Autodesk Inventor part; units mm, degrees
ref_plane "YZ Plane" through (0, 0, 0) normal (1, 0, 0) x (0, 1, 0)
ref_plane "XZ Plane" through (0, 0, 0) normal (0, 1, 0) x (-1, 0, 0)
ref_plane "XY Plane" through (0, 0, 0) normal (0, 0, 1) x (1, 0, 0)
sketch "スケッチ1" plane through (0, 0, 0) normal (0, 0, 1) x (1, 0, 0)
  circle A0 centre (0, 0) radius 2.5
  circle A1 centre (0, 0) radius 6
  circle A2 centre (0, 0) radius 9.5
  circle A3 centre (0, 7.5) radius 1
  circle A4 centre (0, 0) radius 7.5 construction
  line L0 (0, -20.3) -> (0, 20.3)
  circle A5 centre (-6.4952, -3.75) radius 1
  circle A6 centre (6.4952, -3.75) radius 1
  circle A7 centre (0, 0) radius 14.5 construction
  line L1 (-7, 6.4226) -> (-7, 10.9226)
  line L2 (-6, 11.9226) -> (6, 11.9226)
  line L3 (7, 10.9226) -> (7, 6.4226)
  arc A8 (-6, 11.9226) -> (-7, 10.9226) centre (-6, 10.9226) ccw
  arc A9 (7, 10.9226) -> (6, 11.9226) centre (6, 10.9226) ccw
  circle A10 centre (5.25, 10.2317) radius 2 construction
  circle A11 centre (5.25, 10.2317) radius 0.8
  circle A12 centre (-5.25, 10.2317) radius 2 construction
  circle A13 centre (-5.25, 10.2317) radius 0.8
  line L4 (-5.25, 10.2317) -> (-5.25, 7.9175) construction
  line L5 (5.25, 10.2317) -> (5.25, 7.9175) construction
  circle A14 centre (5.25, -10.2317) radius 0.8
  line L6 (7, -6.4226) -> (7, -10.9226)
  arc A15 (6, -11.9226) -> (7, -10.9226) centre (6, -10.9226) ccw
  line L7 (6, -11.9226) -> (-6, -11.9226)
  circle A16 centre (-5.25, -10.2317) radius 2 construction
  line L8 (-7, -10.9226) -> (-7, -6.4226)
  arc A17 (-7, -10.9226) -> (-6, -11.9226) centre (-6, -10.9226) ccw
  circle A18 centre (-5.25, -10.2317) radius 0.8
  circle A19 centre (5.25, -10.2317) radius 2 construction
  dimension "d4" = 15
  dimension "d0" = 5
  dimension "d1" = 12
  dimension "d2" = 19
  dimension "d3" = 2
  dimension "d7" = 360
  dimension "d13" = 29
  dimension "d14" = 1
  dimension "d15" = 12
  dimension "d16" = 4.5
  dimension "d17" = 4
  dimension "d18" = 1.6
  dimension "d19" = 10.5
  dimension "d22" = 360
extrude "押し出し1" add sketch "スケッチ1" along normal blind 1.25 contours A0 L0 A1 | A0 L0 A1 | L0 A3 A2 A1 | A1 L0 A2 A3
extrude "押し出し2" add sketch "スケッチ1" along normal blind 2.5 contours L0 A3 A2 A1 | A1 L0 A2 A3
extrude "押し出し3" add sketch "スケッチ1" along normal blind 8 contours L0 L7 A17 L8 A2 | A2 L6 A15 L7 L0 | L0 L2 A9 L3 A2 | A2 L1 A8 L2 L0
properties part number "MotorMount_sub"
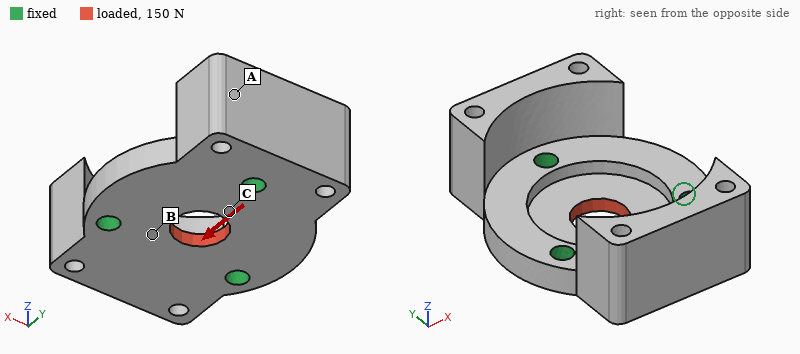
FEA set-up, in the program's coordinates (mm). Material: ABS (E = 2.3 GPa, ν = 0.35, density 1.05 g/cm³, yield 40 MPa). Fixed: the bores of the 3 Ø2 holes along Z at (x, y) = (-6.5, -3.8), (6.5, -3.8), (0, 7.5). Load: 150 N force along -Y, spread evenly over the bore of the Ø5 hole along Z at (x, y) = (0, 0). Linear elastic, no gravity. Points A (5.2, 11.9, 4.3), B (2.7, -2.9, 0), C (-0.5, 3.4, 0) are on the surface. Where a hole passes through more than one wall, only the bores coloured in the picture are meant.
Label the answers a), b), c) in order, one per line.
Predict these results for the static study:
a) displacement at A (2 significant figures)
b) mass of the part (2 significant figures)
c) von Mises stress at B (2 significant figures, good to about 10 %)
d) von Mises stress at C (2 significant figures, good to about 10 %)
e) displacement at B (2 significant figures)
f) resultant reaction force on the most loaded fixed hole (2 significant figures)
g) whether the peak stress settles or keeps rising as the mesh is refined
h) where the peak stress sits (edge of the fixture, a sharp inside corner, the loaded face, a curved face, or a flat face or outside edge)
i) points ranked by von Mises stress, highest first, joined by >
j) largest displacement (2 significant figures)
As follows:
a) 4.1 µm
b) 1.3 g
c) 5.2 MPa
d) 8.5 MPa
e) 15 µm
f) 51 N
g) keeps rising
h) edge of the fixture
i) C > B > A
j) 26 µm
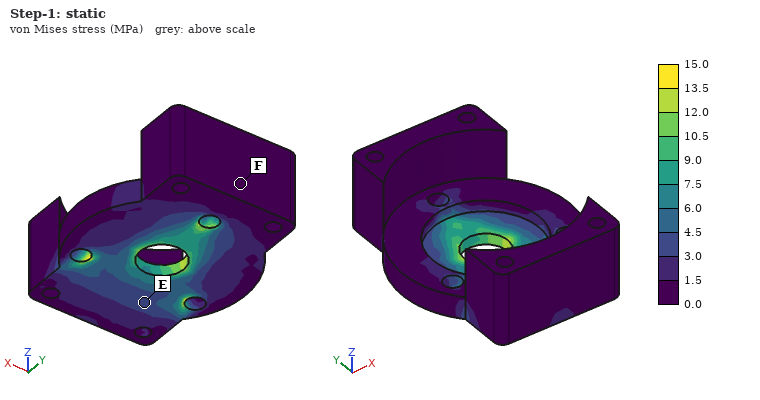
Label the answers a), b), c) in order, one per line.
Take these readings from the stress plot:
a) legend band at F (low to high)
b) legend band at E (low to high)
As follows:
a) 0.0 to 1.5 MPa
b) 3.0 to 4.5 MPa
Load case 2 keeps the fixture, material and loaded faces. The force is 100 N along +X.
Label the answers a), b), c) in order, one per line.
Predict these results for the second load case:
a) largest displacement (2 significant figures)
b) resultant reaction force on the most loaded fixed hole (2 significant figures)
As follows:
a) 17 µm
b) 35 N
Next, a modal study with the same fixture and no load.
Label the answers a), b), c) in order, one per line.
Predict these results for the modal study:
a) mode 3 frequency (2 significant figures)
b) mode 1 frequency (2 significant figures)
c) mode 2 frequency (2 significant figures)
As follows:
a) 7500 Hz
b) 3600 Hz
c) 6400 Hz
